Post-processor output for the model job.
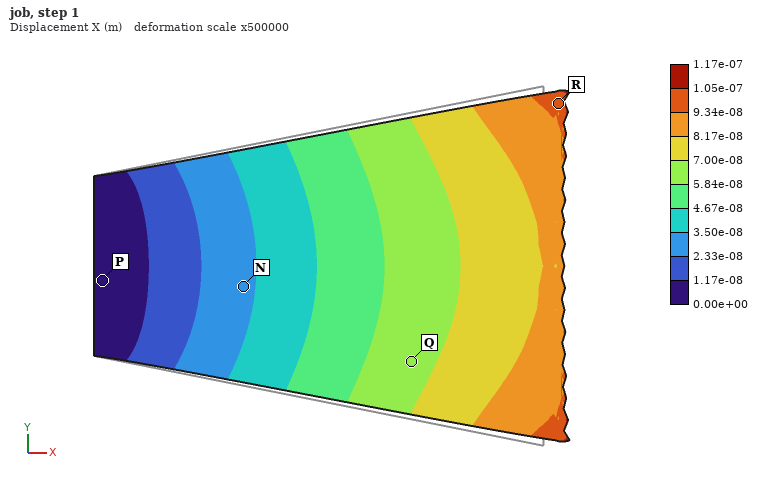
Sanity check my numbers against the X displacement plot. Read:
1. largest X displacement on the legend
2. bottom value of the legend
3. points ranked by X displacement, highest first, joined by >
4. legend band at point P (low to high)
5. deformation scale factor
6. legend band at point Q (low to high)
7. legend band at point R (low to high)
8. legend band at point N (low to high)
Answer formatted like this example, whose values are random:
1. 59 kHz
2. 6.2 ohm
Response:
1. 1.17e-07 m
2. 0.00e+00 m
3. R > Q > N > P
4. 0.00e+00 to 1.17e-08 m
5. 500000
6. 5.84e-08 to 7.00e-08 m
7. 9.34e-08 to 1.05e-07 m
8. 2.33e-08 to 3.50e-08 m
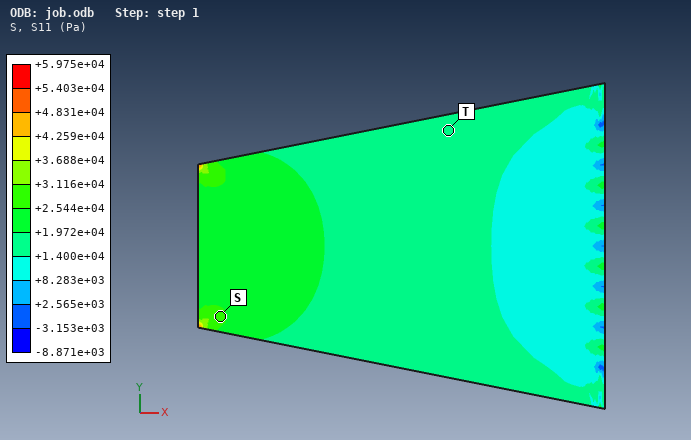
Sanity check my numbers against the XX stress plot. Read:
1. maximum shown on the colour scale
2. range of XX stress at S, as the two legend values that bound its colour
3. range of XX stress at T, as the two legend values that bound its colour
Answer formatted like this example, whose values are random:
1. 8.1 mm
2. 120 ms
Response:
1. +5.975e+04 Pa
2. +2.544e+04 to +3.116e+04 Pa
3. +1.400e+04 to +1.972e+04 Pa
